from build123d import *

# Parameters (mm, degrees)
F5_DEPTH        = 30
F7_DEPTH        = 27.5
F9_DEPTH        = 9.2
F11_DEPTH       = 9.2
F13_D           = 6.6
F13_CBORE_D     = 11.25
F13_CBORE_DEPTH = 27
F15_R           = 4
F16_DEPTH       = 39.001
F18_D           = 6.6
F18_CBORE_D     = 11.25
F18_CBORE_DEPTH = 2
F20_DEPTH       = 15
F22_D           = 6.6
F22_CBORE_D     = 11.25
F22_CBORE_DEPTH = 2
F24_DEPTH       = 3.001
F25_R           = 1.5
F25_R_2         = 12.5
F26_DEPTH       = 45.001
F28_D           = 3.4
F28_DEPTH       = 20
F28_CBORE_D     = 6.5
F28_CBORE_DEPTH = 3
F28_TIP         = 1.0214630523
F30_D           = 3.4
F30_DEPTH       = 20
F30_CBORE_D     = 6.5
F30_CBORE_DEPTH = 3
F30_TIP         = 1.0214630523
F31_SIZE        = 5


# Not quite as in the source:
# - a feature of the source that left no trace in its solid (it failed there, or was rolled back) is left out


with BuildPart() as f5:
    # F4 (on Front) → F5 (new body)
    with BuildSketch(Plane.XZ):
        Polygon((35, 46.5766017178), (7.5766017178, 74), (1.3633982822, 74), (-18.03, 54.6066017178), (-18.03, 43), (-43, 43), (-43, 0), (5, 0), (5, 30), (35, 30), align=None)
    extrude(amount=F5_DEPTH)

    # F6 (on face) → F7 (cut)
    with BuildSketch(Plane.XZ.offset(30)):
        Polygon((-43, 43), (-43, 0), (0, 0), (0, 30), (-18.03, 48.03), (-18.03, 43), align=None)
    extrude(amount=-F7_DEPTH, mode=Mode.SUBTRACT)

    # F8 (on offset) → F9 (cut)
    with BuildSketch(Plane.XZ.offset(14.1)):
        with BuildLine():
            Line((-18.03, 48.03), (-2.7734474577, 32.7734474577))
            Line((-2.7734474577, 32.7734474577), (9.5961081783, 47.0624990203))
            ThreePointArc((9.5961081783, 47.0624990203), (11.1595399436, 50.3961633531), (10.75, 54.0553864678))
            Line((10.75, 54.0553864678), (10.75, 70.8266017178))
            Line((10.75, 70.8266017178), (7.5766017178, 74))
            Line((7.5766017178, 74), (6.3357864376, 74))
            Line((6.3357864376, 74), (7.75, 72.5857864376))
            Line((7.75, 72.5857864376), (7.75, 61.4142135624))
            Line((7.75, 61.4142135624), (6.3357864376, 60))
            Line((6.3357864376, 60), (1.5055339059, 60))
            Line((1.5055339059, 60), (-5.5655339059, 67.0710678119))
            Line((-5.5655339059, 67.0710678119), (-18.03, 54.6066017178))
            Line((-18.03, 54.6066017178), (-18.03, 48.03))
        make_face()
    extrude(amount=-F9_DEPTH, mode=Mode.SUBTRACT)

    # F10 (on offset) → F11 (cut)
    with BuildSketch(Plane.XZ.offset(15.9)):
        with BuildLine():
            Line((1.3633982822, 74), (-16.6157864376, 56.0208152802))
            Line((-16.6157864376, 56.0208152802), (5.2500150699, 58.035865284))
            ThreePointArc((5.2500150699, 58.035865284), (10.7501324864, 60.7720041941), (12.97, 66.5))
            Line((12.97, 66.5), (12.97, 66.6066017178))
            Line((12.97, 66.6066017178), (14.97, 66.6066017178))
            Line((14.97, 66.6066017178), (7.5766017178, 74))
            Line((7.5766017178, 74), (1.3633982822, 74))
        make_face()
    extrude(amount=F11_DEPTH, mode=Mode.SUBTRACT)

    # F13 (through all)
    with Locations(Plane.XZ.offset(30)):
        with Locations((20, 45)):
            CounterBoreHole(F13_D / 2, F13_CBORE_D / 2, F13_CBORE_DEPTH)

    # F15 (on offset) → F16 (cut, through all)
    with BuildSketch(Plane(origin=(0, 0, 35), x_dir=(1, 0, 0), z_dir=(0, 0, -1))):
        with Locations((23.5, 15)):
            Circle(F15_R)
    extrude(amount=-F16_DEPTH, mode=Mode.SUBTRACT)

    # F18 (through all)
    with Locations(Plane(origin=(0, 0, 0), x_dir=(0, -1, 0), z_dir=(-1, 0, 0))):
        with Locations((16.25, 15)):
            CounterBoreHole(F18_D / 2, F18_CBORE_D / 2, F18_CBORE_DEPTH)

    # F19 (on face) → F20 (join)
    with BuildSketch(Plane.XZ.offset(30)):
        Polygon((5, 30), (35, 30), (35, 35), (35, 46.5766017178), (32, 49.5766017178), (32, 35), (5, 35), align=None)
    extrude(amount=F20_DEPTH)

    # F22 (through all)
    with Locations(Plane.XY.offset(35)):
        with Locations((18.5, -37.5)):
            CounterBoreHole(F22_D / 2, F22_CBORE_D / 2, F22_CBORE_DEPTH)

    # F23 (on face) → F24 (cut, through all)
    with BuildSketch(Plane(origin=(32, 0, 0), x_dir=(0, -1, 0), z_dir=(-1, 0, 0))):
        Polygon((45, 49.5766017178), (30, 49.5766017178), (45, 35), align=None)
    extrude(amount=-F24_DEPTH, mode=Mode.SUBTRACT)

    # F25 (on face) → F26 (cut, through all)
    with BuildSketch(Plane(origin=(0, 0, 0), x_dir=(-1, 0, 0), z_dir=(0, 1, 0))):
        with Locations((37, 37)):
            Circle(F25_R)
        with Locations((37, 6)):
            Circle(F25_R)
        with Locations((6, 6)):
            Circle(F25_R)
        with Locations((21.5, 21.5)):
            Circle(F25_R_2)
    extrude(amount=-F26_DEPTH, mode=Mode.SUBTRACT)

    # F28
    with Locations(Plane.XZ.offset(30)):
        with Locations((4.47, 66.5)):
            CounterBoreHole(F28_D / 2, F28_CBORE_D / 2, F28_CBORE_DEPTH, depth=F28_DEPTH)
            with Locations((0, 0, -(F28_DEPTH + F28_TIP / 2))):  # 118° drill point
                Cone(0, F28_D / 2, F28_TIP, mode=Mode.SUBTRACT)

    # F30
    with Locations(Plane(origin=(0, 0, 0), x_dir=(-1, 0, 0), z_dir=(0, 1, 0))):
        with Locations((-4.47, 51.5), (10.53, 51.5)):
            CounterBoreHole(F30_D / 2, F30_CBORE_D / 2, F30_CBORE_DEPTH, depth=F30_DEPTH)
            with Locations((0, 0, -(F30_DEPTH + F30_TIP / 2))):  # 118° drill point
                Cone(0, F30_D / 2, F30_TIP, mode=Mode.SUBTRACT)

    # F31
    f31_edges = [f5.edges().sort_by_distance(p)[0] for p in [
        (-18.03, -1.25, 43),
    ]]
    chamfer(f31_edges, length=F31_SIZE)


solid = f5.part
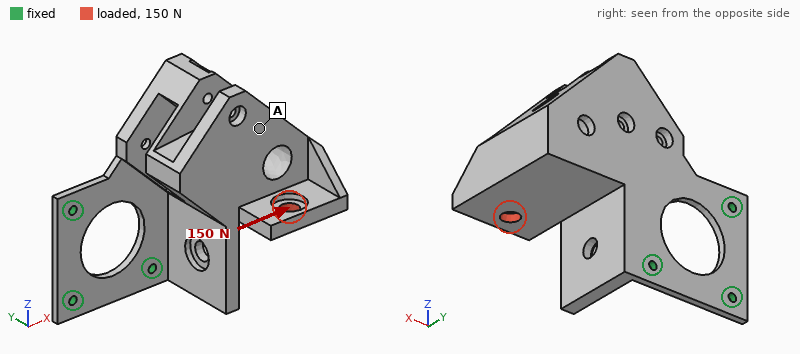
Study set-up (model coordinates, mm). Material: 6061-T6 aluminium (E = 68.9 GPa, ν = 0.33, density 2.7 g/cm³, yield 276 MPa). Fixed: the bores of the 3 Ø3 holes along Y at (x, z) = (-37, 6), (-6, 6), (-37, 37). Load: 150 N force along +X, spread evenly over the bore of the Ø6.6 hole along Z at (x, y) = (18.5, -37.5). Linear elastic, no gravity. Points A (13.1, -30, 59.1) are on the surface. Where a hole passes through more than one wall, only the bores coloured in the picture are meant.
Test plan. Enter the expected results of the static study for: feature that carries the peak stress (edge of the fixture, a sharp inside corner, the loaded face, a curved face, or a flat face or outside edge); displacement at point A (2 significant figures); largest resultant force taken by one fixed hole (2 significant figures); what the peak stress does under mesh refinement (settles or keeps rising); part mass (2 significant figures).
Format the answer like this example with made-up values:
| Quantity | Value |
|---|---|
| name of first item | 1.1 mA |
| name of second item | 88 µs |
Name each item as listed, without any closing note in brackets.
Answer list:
| Quantity | Value |
|---|---|
| feature that carries the peak stress | edge of the fixture |
| displacement at point A | 0.78 mm |
| largest resultant force taken by one fixed hole | 120 N |
| what the peak stress does under mesh refinement | keeps rising |
| part mass | 120 g |
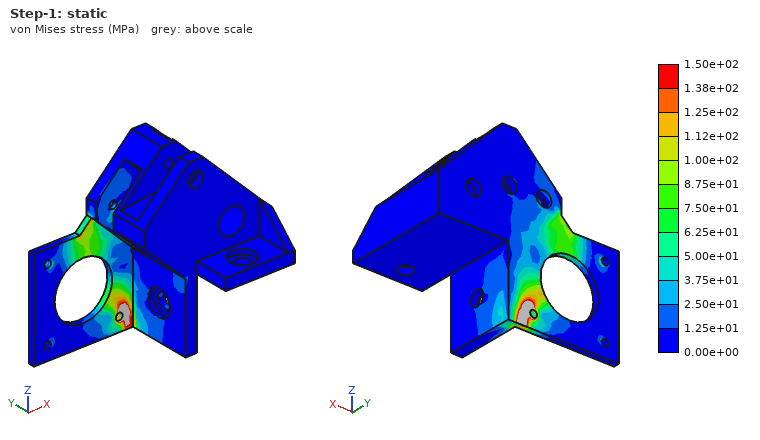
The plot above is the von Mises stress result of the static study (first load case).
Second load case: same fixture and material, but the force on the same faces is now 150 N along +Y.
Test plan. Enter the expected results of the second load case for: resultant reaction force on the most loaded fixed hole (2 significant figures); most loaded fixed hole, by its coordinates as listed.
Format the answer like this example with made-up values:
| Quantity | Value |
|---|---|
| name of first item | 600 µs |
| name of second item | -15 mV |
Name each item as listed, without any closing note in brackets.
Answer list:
| Quantity | Value |
|---|---|
| resultant reaction force on the most loaded fixed hole | 170 N |
| most loaded fixed hole, by its coordinates as listed | (-6, 6) |
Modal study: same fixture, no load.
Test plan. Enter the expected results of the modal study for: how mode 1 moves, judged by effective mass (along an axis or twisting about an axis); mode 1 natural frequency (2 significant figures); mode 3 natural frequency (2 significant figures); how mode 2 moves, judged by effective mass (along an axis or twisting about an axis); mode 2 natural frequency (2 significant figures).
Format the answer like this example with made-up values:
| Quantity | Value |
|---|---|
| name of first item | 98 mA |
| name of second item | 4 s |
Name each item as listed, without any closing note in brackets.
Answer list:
| Quantity | Value |
|---|---|
| how mode 1 moves, judged by effective mass | along Y |
| mode 1 natural frequency | 210 Hz |
| mode 3 natural frequency | 2600 Hz |
| how mode 2 moves, judged by effective mass | along X |
| mode 2 natural frequency | 680 Hz |
